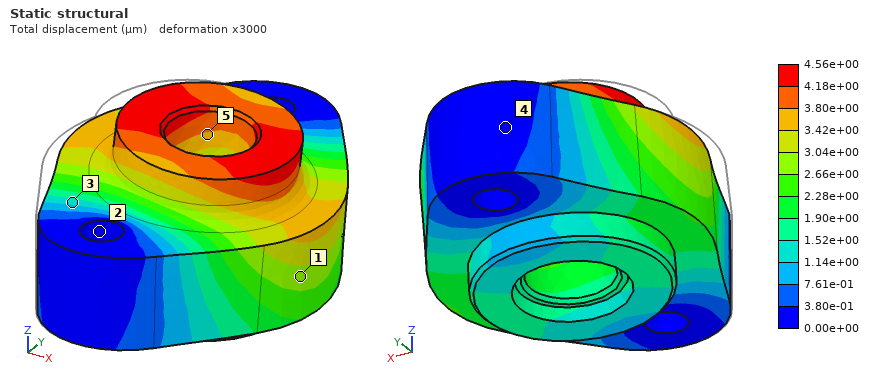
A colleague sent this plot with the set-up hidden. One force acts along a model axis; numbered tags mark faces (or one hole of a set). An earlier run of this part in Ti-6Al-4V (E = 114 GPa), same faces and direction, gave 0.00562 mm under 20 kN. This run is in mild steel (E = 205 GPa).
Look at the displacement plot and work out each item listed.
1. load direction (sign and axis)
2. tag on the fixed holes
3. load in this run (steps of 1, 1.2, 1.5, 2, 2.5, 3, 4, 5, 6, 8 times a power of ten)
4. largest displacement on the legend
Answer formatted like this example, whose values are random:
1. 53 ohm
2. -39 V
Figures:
1. +X
2. 2
3. 30 kN
4. 4.56e+00 µm
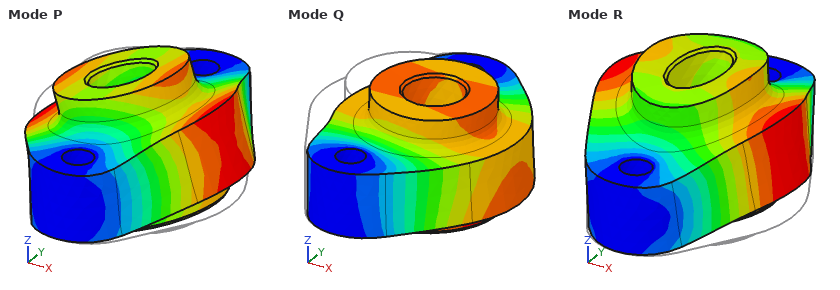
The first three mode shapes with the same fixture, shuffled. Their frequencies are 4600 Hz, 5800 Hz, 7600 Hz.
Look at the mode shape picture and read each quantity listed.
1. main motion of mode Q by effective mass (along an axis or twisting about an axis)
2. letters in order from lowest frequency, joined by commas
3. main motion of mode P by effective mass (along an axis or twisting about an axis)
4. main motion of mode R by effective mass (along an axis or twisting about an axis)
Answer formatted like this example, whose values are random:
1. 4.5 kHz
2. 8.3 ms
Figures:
1. along X
2. P, R, Q
3. twisting about Y
4. along Z
